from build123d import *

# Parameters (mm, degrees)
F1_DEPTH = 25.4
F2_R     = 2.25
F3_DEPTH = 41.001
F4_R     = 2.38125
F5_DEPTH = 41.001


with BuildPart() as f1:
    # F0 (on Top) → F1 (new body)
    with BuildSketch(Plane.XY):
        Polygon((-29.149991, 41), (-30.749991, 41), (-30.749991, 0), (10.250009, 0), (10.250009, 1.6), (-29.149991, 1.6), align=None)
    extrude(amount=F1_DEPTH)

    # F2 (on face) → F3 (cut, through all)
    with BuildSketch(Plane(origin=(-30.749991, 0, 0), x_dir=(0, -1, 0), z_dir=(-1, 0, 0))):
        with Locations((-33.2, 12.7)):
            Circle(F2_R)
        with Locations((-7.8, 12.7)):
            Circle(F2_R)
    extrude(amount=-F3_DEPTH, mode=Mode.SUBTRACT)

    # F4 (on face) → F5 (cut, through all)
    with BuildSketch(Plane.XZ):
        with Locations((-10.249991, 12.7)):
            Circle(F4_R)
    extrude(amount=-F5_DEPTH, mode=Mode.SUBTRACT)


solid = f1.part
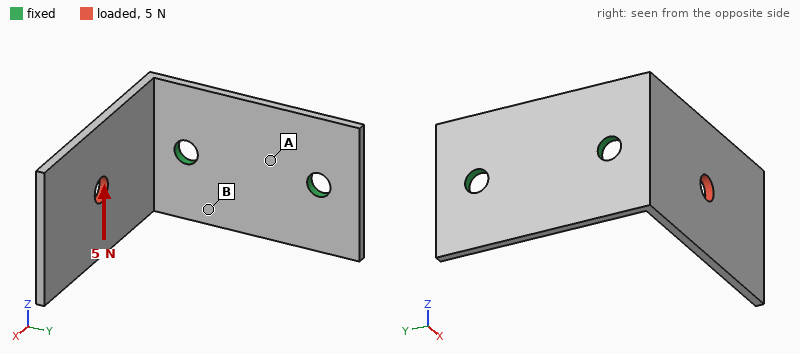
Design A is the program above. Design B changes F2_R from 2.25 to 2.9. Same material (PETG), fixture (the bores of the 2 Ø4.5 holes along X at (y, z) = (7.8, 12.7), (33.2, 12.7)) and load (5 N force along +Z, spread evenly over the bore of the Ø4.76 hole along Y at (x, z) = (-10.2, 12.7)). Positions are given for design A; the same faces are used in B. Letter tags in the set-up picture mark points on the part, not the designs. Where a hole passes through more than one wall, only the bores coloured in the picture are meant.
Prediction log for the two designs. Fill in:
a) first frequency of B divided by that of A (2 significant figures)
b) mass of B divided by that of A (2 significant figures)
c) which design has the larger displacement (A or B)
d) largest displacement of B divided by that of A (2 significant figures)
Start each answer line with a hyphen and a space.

- 1.0
- 0.99
- A
- 0.78
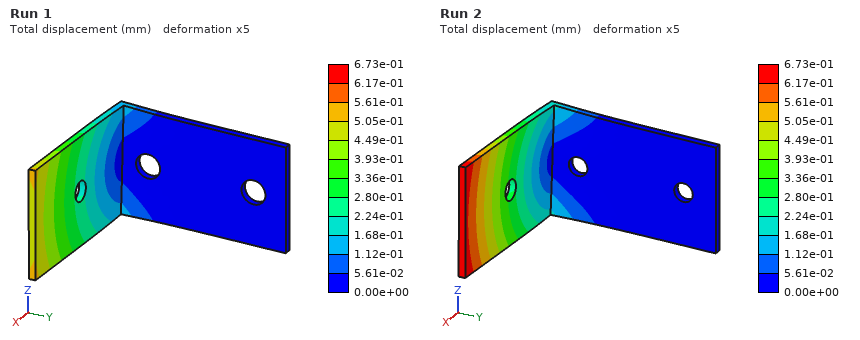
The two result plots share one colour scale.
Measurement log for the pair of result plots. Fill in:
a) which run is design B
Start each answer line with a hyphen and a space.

- Run 1
